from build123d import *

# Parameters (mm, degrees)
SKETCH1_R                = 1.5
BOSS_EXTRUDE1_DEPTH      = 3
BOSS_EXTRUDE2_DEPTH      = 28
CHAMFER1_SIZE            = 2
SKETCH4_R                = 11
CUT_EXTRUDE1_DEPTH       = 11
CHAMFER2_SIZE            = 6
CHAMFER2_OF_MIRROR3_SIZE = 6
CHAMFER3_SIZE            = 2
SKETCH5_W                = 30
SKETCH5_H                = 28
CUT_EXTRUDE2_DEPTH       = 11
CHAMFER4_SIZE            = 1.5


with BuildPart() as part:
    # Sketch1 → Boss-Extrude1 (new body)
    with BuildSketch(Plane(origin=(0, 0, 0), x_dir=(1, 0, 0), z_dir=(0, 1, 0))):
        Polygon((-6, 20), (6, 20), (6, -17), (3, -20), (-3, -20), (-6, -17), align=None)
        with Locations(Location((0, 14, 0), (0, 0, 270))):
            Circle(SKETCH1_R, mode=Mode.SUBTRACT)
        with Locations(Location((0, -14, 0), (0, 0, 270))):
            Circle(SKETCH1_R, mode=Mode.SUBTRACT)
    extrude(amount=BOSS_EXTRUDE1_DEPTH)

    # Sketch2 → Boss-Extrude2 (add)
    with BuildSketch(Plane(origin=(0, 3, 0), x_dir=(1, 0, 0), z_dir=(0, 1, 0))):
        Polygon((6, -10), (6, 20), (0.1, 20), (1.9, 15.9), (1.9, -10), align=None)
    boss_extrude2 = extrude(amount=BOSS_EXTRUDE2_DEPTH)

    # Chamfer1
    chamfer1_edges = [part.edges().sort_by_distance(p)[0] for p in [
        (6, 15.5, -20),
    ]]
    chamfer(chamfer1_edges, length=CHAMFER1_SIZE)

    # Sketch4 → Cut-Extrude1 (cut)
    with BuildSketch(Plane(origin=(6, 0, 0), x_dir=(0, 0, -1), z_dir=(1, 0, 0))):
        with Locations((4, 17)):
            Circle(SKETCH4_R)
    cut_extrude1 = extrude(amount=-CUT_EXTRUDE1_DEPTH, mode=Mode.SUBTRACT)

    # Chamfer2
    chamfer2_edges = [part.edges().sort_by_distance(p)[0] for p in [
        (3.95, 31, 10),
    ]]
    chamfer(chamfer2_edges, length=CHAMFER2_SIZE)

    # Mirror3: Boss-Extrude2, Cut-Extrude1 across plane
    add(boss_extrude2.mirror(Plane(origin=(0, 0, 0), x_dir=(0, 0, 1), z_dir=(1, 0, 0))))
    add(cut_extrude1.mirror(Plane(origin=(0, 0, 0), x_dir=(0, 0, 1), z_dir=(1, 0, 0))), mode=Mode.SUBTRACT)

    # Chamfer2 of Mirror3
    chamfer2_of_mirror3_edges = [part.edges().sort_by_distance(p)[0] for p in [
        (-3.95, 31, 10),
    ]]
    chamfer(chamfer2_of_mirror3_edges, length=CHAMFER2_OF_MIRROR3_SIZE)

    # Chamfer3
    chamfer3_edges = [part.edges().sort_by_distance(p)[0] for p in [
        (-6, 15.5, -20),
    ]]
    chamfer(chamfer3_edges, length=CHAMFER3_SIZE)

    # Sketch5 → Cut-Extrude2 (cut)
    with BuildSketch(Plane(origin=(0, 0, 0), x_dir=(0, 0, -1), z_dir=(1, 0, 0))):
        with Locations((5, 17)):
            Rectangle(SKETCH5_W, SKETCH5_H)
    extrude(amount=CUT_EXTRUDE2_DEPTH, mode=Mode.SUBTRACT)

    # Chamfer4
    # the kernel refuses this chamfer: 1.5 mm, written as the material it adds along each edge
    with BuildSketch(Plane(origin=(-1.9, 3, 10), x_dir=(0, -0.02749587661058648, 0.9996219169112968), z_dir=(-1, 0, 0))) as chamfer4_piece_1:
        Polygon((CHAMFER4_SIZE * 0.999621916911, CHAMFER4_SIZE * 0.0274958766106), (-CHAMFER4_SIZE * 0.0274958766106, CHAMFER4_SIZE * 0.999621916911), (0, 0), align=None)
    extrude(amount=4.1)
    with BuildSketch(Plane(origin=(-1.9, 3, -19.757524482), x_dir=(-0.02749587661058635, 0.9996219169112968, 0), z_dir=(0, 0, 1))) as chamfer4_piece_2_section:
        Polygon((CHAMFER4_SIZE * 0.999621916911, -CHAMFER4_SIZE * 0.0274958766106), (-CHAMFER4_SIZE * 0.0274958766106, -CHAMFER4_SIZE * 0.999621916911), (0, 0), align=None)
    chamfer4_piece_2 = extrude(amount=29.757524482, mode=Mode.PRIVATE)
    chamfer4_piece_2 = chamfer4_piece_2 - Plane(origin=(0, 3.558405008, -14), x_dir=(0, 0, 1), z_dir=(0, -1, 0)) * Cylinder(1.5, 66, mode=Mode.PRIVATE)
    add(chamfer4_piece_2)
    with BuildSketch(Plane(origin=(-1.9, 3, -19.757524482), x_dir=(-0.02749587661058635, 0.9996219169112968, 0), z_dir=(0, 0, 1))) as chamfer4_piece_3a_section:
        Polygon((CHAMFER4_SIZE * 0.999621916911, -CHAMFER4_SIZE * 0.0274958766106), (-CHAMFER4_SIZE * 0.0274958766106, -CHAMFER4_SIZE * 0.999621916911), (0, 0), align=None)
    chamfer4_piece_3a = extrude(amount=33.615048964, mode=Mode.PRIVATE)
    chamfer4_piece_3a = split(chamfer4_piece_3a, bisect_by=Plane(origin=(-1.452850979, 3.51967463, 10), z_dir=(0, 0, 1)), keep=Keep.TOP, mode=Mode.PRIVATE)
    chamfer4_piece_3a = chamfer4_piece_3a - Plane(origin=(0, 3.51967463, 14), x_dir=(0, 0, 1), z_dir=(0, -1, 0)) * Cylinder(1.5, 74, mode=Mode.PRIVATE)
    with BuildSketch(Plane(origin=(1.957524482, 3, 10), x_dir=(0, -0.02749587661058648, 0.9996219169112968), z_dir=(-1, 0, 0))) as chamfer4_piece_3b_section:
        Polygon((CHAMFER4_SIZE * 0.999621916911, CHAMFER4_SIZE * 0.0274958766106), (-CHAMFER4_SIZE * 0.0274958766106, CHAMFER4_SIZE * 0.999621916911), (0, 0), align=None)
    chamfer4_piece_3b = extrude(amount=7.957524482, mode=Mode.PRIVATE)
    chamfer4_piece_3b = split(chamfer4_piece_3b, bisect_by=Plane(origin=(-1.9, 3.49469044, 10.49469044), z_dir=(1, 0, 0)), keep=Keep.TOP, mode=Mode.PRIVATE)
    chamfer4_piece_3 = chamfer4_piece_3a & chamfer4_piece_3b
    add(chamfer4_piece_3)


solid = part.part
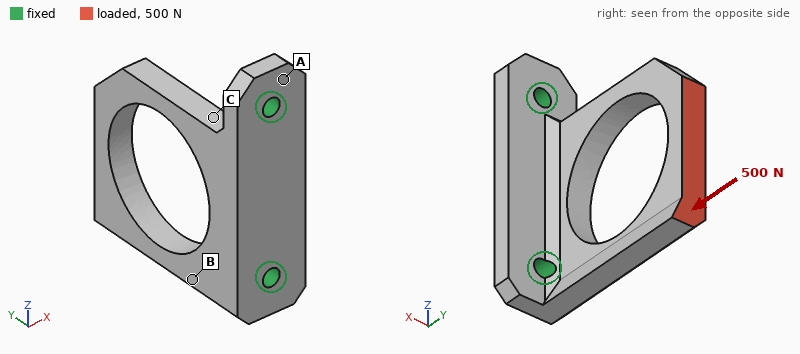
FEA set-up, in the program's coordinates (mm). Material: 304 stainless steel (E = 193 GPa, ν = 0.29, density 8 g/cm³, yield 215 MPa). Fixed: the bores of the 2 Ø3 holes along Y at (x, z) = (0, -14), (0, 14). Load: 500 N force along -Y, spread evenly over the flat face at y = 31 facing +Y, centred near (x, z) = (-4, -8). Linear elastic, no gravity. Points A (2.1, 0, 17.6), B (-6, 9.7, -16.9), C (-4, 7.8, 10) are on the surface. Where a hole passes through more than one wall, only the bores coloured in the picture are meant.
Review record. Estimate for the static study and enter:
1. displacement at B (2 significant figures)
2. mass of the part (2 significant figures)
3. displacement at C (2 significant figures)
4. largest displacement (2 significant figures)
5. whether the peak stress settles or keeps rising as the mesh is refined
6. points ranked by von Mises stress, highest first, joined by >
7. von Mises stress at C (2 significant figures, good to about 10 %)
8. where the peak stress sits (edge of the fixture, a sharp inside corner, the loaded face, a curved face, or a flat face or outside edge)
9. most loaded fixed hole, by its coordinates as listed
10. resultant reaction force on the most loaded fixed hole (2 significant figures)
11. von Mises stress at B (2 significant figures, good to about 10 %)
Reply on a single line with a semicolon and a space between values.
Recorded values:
4.0 µm; 26 g; 2.8 µm; 13 µm; keeps rising; C > B > A; 30 MPa; edge of the fixture; (0, -14); 350 N; 19 MPa
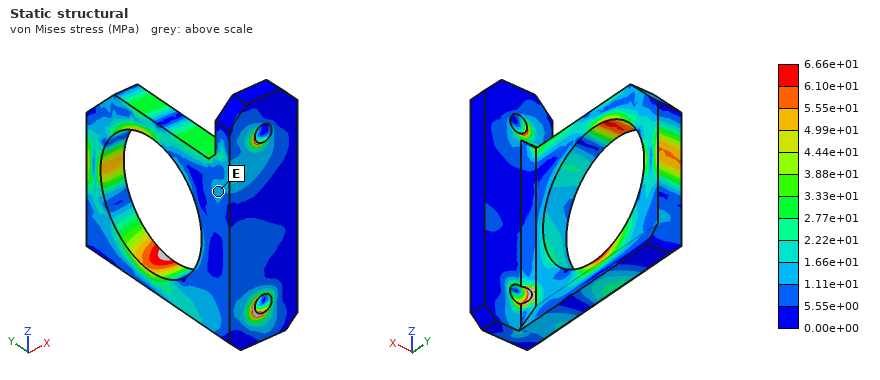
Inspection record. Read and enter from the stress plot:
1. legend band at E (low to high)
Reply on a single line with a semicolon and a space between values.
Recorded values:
1.11e+01 to 1.66e+01 MPa
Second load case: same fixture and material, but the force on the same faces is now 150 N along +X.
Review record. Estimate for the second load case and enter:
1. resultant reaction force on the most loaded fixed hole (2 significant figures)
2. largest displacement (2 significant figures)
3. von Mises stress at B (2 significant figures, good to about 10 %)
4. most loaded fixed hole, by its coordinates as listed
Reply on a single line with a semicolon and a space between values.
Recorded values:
130 N; 0.10 mm; 100 MPa; (0, -14)
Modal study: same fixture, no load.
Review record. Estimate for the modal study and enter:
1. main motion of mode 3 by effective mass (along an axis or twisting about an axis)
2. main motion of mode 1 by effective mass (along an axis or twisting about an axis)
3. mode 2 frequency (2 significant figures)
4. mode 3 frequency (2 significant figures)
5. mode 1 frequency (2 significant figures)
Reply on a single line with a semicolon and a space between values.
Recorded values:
along Z; along X; 6300 Hz; 7700 Hz; 3000 Hz
